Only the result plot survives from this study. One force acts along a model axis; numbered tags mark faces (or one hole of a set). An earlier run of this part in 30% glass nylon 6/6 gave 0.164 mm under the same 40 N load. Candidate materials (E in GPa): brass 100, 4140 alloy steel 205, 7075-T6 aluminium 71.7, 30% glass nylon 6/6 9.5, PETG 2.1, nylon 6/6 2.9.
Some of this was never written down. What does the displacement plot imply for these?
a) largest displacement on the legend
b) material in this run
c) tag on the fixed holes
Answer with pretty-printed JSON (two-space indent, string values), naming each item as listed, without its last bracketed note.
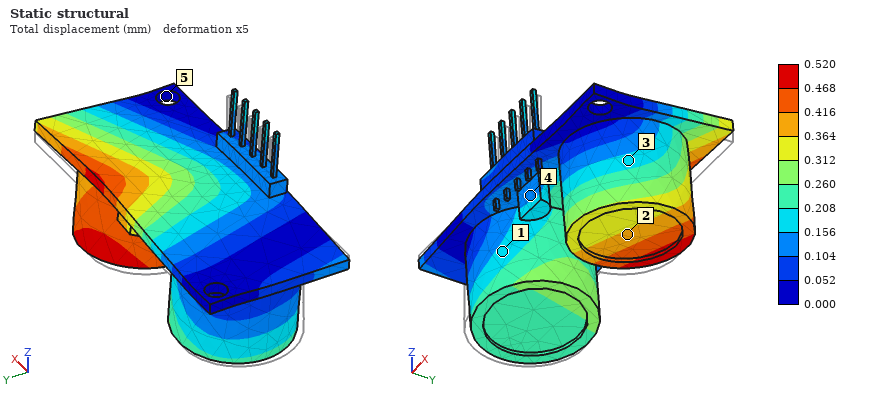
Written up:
{
  "largest displacement on the legend": "0.520 mm",
  "material in this run": "nylon 6/6",
  "tag on the fixed holes": "5"
}
